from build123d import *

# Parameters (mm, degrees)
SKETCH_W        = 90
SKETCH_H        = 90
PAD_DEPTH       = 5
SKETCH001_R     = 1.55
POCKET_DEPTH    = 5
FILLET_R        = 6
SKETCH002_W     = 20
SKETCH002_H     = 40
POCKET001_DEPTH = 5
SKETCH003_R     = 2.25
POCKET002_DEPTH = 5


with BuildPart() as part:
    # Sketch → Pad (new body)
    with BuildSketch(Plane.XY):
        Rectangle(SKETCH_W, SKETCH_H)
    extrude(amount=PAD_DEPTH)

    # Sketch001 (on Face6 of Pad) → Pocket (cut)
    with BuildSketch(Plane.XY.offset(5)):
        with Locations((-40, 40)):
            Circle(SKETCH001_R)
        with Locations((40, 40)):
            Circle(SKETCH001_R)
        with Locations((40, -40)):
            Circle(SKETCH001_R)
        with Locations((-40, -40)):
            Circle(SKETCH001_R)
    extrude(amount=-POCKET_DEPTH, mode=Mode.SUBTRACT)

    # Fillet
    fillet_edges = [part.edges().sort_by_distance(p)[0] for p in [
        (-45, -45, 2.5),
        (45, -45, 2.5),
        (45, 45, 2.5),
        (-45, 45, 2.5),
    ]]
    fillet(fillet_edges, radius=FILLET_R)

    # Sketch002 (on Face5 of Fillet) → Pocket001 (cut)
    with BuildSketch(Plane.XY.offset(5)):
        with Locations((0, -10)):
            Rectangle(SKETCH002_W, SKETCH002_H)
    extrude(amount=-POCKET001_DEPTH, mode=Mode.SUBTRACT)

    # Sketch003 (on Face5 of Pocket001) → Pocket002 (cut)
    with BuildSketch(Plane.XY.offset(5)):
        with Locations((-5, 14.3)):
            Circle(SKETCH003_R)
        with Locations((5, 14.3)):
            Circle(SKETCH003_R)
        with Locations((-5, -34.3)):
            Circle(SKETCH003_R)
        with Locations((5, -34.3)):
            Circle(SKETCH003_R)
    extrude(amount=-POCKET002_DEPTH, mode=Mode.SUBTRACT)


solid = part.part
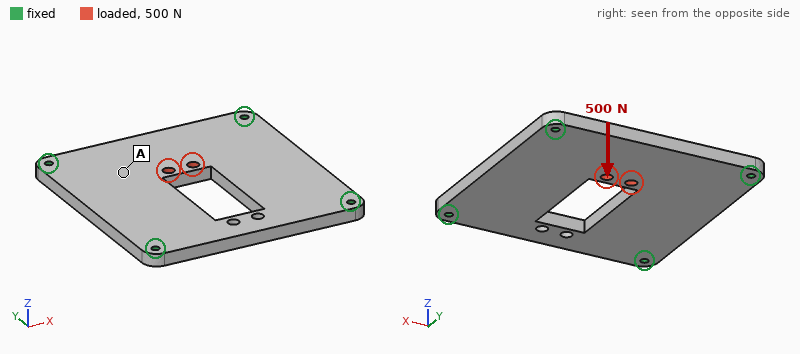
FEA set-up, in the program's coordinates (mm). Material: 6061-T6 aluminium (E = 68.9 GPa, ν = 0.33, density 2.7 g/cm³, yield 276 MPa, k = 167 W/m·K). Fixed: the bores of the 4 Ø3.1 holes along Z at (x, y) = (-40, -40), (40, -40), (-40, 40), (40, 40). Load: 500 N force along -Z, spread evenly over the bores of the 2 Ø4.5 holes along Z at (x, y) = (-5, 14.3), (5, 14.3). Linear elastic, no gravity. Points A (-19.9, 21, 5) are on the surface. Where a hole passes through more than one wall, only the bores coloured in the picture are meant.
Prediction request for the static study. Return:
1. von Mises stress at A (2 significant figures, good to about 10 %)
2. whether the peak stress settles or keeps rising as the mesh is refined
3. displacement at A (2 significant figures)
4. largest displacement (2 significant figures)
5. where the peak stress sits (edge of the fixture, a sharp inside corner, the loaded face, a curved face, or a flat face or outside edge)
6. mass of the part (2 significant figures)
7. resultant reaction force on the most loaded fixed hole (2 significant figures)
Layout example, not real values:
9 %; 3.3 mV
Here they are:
13 MPa; keeps rising; 0.058 mm; 0.12 mm; edge of the fixture; 97 g; 180 N
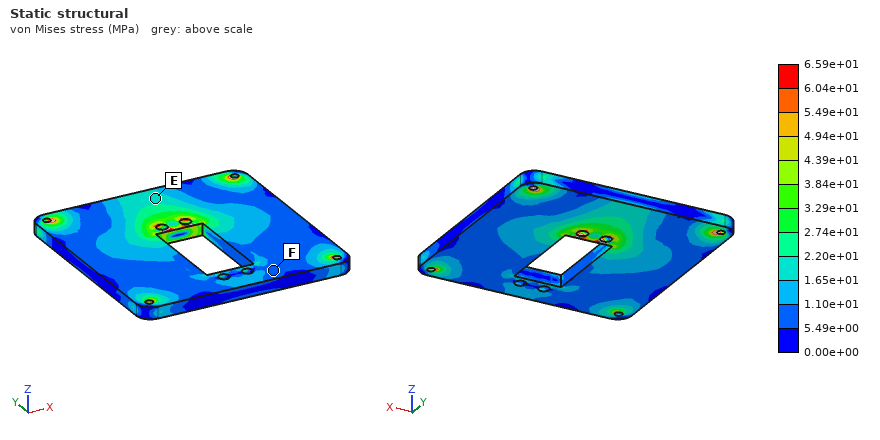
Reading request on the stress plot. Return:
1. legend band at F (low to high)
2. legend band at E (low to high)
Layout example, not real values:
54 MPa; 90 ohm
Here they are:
5.49e+00 to 1.10e+01 MPa; 1.65e+01 to 2.20e+01 MPa
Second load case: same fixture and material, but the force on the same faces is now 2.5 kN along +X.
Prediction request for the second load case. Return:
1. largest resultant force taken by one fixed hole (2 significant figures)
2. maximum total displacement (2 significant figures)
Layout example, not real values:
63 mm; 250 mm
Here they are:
1.1 kN; 12 µm
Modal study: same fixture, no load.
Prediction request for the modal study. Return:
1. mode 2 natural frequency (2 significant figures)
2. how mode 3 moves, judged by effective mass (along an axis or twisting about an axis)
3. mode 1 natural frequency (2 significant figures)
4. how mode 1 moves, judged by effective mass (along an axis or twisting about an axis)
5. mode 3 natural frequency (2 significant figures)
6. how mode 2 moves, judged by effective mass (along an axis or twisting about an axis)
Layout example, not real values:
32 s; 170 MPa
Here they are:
3800 Hz; twisting about X; 2300 Hz; along Z; 4200 Hz; twisting about Y
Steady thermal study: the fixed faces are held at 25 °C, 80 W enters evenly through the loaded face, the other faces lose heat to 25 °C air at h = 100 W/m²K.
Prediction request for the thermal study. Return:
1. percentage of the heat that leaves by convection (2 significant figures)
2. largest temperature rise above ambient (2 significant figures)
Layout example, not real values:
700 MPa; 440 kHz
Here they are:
34 %; 68 K
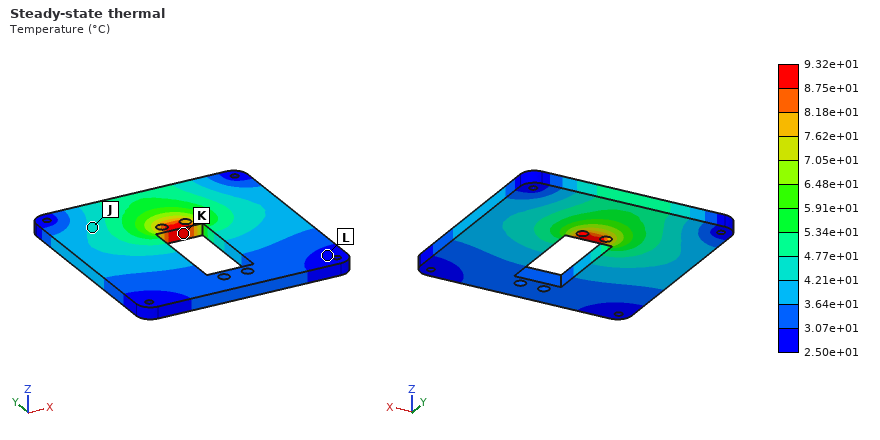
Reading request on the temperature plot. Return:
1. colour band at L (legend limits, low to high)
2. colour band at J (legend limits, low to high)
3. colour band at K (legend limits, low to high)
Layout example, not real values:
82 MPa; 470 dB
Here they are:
2.50e+01 to 3.07e+01 °C; 4.21e+01 to 4.77e+01 °C; 8.75e+01 to 9.32e+01 °C
